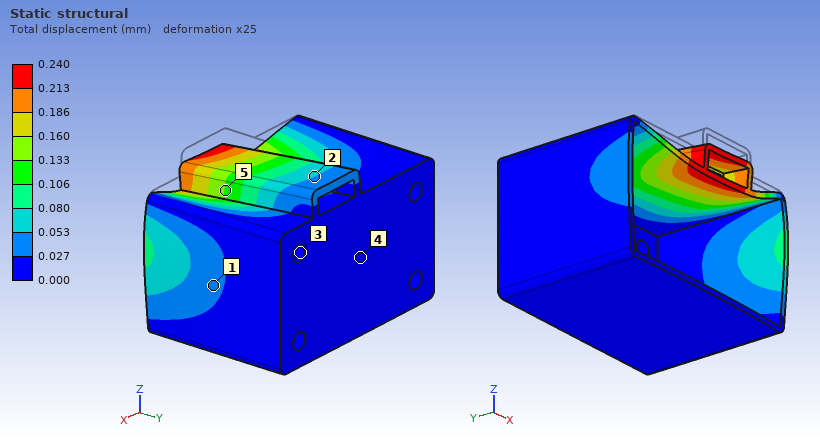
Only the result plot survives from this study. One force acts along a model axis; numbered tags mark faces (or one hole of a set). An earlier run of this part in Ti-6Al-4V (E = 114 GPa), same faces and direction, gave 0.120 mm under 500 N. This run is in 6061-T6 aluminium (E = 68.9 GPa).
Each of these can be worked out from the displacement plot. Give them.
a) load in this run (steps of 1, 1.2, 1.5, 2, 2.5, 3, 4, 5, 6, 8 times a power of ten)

600 N
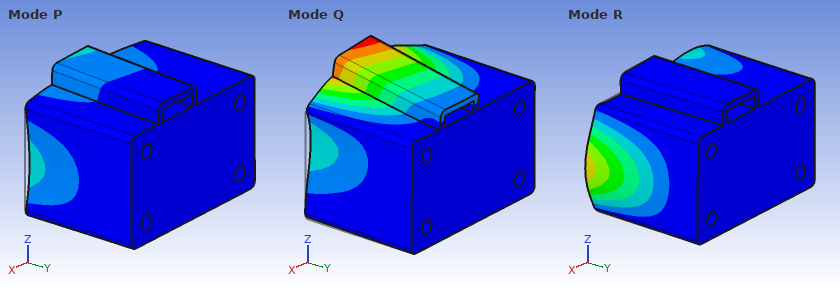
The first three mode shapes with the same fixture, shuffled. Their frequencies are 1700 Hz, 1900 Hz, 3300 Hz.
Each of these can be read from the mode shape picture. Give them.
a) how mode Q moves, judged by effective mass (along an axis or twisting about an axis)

along Z
